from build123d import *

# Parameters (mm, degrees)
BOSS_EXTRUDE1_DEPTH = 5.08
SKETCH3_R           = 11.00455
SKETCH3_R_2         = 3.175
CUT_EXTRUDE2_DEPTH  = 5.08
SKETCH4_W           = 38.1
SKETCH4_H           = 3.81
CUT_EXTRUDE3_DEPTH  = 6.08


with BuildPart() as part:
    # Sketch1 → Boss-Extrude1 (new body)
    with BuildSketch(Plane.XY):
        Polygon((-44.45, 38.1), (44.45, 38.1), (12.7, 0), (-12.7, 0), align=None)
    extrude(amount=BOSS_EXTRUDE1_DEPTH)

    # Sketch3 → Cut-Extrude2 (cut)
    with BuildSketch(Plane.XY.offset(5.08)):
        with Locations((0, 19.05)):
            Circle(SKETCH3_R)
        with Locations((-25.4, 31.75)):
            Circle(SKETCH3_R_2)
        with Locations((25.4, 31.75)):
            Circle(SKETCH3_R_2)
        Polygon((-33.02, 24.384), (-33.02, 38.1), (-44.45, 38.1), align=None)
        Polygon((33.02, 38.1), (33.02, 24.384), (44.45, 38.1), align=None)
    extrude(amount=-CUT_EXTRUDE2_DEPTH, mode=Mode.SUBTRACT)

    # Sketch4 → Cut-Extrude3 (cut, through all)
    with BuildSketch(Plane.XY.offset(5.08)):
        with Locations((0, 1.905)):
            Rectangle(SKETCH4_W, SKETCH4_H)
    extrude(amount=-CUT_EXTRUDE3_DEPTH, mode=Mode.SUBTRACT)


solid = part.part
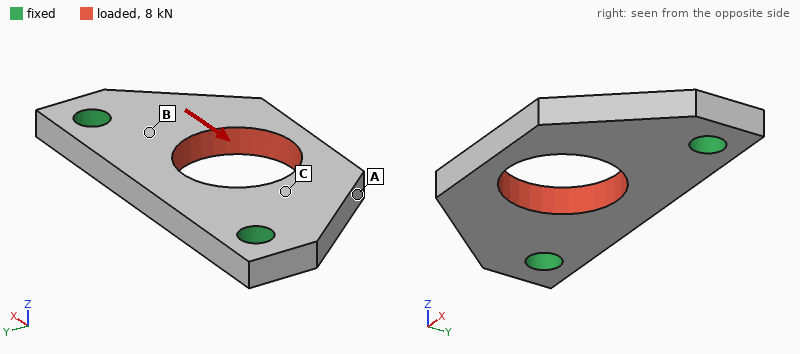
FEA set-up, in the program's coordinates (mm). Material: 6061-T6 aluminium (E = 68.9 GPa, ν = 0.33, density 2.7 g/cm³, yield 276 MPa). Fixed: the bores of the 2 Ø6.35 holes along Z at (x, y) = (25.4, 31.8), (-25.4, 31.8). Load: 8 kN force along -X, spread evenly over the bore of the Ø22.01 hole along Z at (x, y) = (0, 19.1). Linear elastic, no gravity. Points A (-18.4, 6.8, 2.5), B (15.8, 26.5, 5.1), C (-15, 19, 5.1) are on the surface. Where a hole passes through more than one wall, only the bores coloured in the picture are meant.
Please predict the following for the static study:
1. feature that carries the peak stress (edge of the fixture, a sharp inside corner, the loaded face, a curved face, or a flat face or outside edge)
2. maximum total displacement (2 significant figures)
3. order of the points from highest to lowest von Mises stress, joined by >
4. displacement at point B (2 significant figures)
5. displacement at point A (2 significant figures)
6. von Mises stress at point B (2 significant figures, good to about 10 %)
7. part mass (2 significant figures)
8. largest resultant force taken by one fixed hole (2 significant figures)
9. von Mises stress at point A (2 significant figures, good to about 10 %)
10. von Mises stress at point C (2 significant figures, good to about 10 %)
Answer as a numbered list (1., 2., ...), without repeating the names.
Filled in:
1. edge of the fixture
2. 59 µm
3. C > B > A
4. 13 µm
5. 51 µm
6. 33 MPa
7. 20 g
8. 4.2 kN
9. 15 MPa
10. 55 MPa
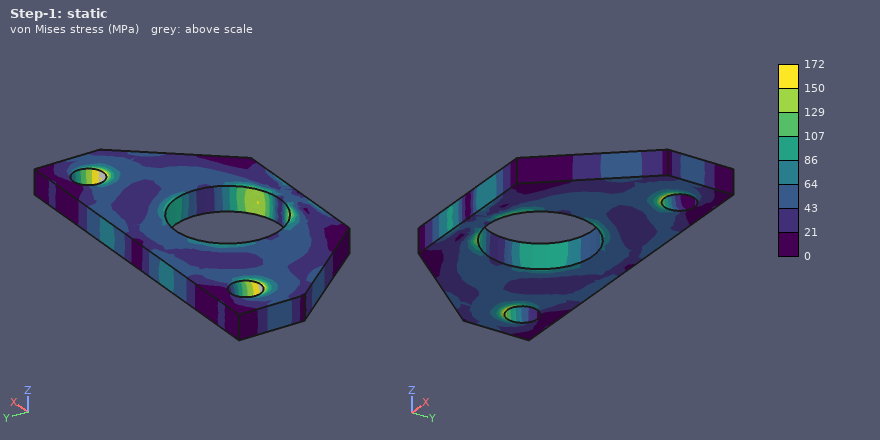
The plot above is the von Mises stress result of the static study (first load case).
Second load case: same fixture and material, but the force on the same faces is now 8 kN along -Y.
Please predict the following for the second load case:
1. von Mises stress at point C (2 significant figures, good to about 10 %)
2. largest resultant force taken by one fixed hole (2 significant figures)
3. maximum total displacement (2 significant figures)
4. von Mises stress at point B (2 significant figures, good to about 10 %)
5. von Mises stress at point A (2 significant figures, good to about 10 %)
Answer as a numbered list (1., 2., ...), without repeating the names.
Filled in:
1. 59 MPa
2. 4.2 kN
3. 43 µm
4. 53 MPa
5. 23 MPa
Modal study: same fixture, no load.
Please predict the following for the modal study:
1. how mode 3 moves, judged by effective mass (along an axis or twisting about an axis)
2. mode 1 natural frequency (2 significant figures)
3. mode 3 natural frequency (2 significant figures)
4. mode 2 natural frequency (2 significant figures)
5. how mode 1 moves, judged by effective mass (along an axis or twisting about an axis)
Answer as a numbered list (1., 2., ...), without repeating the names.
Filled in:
1. along Z
2. 5100 Hz
3. 12 kHz
4. 10 kHz
5. along Z
